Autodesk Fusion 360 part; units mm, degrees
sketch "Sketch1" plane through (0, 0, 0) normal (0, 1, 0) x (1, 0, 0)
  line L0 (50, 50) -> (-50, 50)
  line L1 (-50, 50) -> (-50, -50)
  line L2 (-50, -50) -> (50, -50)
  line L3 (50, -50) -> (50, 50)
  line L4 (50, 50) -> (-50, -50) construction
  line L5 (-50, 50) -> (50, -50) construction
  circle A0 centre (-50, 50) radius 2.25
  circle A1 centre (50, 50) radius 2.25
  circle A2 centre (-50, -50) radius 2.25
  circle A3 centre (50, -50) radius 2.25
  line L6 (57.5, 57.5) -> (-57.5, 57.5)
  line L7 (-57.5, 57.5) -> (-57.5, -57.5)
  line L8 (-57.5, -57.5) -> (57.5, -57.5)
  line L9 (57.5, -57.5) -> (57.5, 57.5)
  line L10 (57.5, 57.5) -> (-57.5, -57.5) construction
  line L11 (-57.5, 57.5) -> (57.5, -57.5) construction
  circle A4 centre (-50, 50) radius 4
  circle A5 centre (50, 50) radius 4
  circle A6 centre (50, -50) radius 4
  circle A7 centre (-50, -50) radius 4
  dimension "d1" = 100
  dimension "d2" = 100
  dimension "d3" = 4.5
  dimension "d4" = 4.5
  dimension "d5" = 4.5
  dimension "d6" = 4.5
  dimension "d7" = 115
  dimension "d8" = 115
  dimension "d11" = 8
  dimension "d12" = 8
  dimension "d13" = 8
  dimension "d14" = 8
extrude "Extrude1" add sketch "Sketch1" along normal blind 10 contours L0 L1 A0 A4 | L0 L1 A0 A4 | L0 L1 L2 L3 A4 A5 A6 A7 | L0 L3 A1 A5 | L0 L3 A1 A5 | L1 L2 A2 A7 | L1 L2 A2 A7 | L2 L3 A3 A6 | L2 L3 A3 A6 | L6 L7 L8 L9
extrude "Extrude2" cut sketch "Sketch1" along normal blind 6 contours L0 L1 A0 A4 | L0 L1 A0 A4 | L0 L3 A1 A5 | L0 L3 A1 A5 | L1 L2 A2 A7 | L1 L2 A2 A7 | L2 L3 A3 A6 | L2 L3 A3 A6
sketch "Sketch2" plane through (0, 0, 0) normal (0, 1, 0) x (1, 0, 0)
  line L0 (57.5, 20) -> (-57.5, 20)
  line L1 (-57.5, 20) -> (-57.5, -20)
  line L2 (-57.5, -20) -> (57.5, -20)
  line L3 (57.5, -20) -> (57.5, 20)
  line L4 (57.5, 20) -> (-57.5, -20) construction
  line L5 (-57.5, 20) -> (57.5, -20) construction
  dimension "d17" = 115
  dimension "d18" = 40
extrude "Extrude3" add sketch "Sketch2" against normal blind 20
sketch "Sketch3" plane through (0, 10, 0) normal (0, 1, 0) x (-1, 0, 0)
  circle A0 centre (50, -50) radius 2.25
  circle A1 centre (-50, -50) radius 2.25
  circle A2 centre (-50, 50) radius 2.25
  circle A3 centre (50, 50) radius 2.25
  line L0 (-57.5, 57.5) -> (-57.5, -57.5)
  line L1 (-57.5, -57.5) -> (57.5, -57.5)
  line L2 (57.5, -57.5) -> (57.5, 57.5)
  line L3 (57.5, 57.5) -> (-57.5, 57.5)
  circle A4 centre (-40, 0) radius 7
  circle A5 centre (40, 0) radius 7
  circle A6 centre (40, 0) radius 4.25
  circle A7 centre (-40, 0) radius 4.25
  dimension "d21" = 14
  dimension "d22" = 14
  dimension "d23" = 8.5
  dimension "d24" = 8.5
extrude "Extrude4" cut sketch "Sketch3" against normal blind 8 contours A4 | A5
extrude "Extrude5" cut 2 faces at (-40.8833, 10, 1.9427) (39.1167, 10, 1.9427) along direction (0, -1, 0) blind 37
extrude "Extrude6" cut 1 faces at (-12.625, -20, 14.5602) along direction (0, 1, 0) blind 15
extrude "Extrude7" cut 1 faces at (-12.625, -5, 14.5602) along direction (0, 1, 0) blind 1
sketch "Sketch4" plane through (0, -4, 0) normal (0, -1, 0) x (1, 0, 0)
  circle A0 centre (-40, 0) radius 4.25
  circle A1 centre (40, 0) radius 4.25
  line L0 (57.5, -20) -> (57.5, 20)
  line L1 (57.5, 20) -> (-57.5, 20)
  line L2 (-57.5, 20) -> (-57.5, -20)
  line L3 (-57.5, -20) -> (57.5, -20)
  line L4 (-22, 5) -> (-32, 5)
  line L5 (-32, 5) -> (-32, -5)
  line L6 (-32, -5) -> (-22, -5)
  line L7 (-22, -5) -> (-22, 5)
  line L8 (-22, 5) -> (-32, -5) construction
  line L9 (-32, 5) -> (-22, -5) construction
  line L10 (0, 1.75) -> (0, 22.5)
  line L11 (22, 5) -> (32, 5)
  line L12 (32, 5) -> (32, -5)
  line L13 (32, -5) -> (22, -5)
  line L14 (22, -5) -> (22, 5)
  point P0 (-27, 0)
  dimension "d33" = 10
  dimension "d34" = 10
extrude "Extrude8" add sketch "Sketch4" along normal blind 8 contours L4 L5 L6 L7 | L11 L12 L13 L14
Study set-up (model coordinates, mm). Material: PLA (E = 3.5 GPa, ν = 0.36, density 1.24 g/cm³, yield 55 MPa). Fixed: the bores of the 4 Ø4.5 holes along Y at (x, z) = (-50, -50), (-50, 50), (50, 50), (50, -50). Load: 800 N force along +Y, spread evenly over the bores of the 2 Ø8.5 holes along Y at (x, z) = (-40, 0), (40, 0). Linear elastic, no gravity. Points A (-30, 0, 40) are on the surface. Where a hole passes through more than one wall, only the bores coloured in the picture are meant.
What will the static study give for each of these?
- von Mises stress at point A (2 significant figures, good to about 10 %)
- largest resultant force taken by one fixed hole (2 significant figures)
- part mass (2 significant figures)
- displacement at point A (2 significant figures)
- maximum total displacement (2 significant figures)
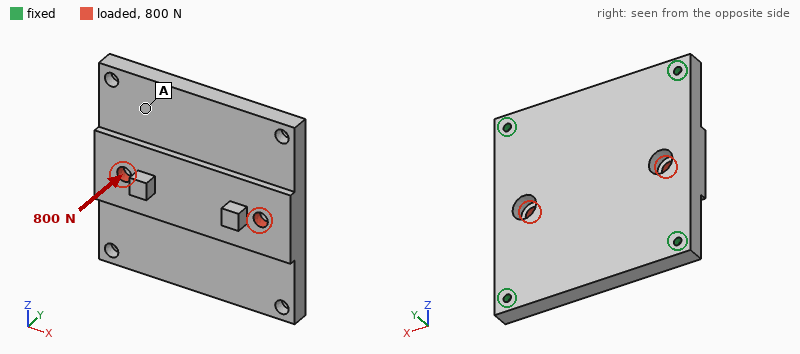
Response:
1.9 MPa
400 N
180 g
0.099 mm
0.24 mm
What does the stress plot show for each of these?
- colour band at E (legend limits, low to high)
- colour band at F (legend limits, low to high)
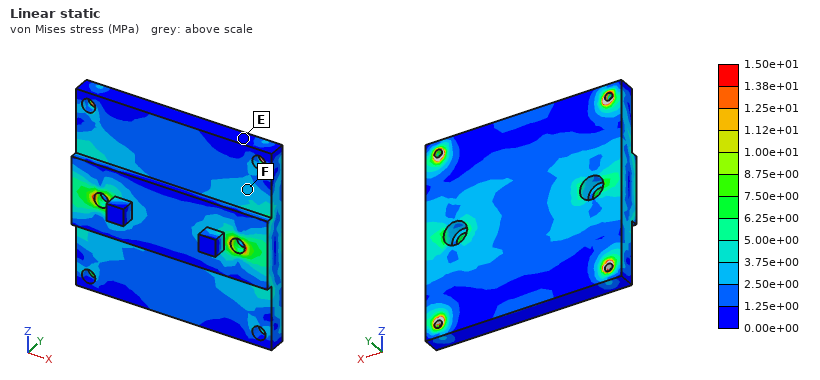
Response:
0.00e+00 to 1.25e+00 MPa
2.50e+00 to 3.75e+00 MPa
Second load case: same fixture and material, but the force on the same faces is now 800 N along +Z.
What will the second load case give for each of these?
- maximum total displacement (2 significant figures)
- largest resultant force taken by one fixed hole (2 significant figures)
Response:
22 µm
210 N
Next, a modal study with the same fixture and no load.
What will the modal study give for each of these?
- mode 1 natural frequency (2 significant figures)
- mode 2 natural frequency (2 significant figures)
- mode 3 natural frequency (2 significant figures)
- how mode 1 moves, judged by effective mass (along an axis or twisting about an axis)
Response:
870 Hz
1500 Hz
1500 Hz
along Y
